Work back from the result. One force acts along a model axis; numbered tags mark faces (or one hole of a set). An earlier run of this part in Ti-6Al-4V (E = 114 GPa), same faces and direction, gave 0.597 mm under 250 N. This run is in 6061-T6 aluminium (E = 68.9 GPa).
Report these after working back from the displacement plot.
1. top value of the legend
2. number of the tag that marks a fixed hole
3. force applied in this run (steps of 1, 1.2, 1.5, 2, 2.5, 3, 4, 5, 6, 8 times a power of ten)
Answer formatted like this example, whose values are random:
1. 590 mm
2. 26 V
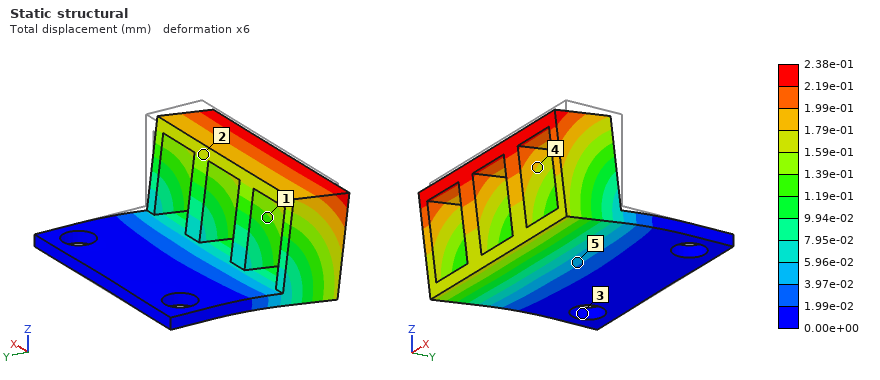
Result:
1. 2.38e-01 mm
2. 3
3. 60 N
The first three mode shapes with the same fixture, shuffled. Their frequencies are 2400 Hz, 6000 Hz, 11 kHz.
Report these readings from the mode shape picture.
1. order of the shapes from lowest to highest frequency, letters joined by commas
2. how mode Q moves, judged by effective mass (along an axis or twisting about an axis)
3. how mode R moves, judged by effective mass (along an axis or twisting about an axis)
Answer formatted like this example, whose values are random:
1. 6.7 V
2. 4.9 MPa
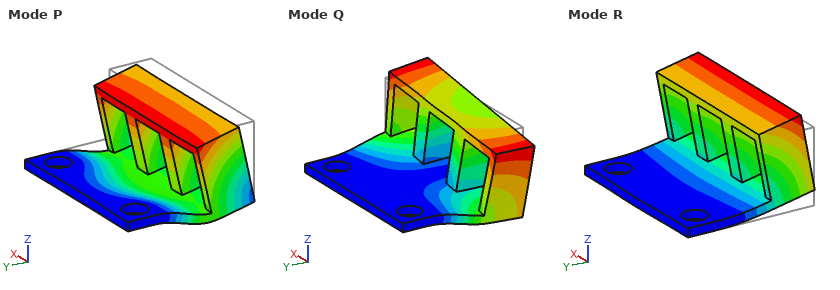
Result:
1. R, Q, P
2. along X
3. along Z
